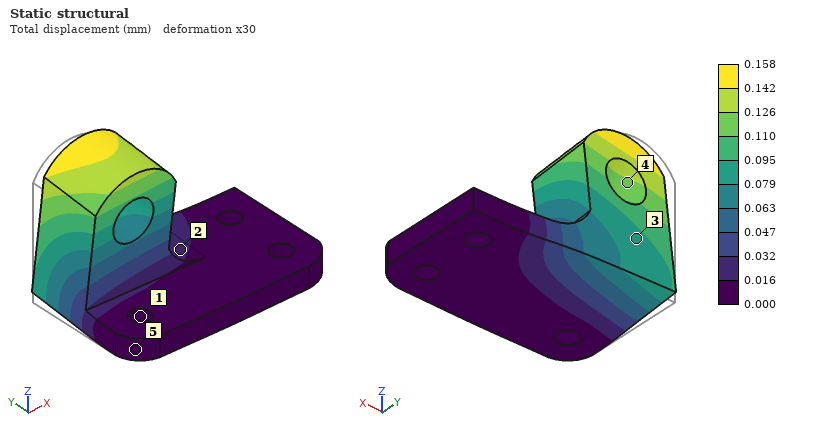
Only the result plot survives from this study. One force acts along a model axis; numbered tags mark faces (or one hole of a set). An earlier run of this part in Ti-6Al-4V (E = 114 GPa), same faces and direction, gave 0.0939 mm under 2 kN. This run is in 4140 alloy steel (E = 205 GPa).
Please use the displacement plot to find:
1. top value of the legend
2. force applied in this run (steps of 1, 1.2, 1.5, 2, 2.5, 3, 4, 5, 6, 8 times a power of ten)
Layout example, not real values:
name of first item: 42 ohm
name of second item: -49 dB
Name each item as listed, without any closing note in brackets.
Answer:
top value of the legend: 0.158 mm
force applied in this run: 6 kN
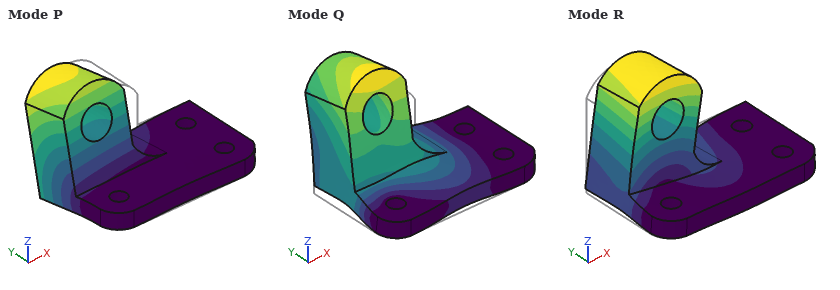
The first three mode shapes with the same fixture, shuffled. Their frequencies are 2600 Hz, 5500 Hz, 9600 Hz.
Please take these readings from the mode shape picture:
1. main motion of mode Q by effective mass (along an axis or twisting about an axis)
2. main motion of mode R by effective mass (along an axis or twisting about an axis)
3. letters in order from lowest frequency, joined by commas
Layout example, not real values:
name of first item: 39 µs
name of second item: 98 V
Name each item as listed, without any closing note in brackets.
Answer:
main motion of mode Q by effective mass: along Z
main motion of mode R by effective mass: along X
letters in order from lowest frequency, joined by commas: P, R, Q
